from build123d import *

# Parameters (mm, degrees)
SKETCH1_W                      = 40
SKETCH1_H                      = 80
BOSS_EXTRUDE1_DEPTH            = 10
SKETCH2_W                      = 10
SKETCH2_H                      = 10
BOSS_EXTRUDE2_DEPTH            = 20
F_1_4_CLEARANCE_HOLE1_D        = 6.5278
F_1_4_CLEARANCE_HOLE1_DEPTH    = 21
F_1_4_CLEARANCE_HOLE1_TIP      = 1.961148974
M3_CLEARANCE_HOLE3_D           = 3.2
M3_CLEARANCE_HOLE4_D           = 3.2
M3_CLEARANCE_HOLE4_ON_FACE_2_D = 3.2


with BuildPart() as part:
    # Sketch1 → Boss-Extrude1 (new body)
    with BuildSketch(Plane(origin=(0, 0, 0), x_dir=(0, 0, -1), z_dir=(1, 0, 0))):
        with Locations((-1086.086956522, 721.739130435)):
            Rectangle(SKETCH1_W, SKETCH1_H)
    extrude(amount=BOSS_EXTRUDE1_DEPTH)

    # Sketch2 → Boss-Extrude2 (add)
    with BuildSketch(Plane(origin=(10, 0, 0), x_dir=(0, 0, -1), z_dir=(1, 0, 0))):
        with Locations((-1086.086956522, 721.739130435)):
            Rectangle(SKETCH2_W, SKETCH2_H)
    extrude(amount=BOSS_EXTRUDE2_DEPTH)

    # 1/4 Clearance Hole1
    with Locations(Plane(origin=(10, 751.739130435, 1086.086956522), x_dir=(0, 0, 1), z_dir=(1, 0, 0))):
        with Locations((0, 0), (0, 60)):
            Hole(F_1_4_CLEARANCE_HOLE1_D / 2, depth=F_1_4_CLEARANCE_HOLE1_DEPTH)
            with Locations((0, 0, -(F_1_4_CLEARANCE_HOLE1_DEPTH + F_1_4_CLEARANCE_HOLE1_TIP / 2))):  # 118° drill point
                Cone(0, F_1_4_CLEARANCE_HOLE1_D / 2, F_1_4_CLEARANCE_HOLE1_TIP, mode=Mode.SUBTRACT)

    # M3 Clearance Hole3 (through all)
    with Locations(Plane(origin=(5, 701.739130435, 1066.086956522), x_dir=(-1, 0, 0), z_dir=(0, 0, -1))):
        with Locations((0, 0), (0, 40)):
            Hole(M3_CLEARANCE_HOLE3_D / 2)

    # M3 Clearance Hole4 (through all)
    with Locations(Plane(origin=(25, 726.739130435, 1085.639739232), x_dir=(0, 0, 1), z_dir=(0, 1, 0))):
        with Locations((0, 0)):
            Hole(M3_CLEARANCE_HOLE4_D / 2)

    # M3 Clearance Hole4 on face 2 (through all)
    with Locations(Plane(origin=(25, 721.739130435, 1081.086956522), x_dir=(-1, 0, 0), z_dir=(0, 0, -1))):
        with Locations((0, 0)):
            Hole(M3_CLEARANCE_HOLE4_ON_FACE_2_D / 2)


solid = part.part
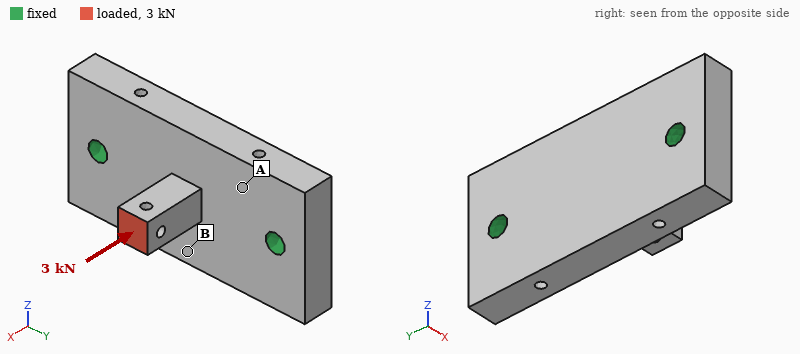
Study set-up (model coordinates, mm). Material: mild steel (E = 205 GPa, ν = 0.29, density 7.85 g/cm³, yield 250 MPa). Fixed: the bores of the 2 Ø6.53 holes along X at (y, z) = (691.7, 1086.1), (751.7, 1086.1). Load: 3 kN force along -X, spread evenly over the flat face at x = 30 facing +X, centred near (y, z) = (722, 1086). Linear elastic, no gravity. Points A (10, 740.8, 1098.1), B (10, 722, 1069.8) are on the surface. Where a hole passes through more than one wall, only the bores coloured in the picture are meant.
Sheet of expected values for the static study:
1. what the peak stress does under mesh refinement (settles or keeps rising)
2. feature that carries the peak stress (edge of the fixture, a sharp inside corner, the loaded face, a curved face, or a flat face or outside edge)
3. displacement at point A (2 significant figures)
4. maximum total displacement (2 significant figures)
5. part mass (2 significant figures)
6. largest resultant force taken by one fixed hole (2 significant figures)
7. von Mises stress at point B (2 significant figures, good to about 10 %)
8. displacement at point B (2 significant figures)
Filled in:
keeps rising
a sharp inside corner
3.5 µm
12 µm
260 g
1.5 kN
22 MPa
7.0 µm
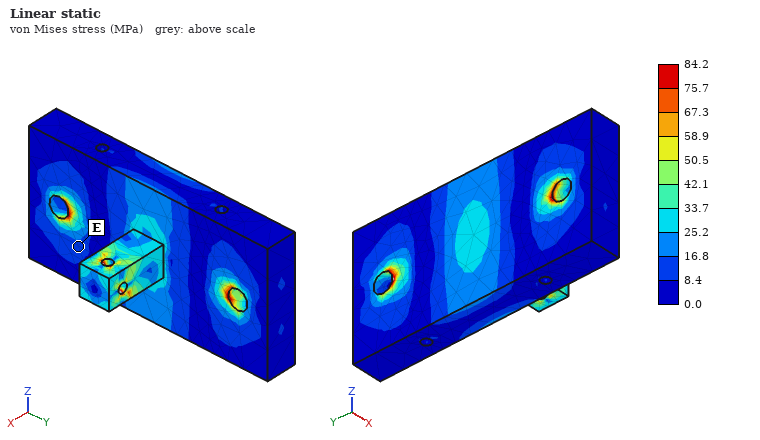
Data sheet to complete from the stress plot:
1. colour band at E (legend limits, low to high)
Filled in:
8.4 to 16.8 MPa
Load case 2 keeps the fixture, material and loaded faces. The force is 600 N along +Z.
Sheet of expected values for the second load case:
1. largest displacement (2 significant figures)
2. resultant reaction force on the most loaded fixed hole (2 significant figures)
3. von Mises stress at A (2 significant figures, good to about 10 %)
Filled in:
23 µm
300 N
8.2 MPa
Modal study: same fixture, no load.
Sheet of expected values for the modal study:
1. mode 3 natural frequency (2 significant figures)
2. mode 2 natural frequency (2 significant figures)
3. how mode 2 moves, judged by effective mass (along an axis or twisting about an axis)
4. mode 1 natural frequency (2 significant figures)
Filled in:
14 kHz
9700 Hz
along X
9100 Hz
